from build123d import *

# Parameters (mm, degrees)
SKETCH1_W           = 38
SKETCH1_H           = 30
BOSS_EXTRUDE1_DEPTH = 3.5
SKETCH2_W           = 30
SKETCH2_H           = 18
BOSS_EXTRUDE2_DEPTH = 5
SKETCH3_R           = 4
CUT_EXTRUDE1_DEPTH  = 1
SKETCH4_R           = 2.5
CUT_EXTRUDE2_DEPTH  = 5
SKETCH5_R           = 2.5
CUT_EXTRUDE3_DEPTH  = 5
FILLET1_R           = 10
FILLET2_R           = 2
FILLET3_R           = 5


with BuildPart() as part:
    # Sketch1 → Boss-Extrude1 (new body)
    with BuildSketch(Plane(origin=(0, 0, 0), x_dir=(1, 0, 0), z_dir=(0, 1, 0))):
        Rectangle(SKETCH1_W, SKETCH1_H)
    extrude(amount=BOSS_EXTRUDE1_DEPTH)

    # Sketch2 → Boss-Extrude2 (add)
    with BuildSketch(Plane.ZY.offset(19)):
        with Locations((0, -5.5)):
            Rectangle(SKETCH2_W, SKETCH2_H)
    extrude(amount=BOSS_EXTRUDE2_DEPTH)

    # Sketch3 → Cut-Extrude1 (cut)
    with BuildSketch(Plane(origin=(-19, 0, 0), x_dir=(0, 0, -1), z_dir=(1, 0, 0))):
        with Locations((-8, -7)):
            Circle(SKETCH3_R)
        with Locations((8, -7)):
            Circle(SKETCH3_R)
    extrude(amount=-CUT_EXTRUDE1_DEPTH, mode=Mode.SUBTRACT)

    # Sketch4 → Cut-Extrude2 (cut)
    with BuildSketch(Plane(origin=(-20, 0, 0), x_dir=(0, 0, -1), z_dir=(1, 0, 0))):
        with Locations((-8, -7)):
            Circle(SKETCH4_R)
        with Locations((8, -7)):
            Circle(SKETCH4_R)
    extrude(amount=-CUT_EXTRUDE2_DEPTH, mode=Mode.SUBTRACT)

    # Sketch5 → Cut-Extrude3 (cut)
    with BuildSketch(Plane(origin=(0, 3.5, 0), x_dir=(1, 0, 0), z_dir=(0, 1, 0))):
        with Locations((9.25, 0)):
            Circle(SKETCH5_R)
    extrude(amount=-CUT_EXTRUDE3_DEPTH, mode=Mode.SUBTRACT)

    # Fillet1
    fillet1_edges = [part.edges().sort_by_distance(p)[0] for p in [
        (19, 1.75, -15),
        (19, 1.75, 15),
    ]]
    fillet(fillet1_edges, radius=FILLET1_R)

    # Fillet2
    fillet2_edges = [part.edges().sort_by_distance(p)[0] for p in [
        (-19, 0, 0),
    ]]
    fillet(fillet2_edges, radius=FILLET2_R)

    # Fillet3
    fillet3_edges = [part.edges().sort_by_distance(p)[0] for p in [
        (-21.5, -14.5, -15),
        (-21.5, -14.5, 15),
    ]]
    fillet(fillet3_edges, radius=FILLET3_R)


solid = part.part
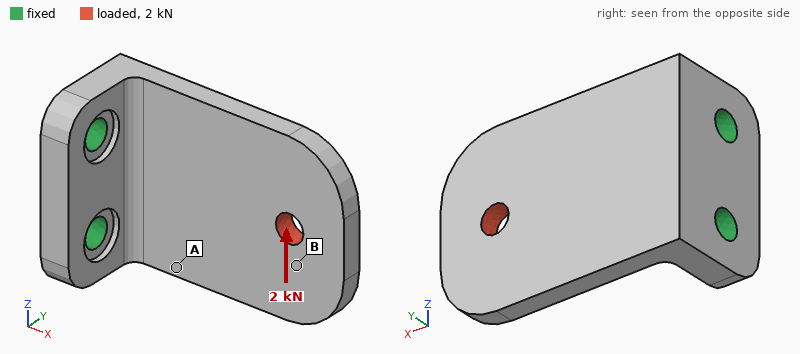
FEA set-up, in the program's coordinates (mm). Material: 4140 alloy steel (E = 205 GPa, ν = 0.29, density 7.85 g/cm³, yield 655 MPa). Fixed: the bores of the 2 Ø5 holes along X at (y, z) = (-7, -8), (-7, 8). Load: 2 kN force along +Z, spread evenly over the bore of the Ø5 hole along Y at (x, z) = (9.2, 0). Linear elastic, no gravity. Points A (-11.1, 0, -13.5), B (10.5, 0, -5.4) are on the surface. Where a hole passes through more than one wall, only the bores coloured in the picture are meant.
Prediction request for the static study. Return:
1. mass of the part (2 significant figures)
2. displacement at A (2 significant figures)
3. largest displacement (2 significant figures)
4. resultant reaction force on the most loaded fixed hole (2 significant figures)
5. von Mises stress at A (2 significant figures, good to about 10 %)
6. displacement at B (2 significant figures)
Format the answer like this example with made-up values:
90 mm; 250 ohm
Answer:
49 g; 0.043 mm; 0.10 mm; 3.4 kN; 120 MPa; 0.084 mm
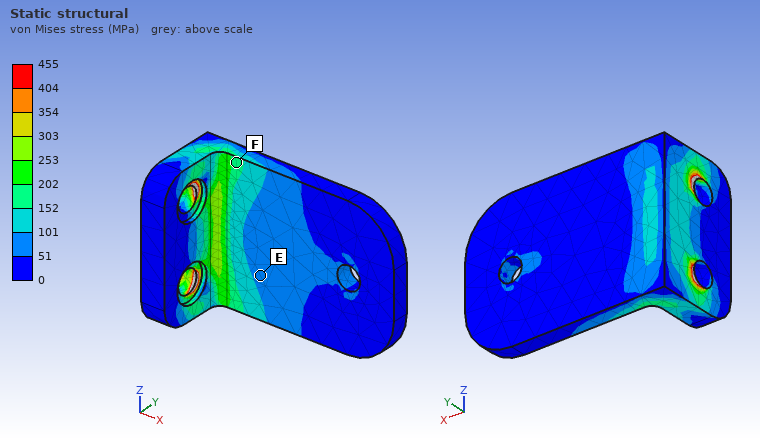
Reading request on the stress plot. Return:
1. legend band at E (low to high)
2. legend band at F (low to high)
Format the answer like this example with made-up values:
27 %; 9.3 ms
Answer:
51 to 101 MPa; 152 to 202 MPa
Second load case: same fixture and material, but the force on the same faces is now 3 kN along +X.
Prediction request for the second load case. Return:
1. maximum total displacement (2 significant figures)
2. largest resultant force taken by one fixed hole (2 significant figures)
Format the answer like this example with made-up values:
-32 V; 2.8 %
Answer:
87 µm; 1.5 kN
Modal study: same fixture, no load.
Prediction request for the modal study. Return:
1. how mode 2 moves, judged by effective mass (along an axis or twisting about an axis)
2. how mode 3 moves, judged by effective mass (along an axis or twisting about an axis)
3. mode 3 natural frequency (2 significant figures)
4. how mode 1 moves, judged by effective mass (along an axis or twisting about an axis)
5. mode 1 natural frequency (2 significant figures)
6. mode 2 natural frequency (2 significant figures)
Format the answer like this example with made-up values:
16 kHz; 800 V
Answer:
along Z; along Z; 6800 Hz; along Y; 1800 Hz; 5300 Hz
